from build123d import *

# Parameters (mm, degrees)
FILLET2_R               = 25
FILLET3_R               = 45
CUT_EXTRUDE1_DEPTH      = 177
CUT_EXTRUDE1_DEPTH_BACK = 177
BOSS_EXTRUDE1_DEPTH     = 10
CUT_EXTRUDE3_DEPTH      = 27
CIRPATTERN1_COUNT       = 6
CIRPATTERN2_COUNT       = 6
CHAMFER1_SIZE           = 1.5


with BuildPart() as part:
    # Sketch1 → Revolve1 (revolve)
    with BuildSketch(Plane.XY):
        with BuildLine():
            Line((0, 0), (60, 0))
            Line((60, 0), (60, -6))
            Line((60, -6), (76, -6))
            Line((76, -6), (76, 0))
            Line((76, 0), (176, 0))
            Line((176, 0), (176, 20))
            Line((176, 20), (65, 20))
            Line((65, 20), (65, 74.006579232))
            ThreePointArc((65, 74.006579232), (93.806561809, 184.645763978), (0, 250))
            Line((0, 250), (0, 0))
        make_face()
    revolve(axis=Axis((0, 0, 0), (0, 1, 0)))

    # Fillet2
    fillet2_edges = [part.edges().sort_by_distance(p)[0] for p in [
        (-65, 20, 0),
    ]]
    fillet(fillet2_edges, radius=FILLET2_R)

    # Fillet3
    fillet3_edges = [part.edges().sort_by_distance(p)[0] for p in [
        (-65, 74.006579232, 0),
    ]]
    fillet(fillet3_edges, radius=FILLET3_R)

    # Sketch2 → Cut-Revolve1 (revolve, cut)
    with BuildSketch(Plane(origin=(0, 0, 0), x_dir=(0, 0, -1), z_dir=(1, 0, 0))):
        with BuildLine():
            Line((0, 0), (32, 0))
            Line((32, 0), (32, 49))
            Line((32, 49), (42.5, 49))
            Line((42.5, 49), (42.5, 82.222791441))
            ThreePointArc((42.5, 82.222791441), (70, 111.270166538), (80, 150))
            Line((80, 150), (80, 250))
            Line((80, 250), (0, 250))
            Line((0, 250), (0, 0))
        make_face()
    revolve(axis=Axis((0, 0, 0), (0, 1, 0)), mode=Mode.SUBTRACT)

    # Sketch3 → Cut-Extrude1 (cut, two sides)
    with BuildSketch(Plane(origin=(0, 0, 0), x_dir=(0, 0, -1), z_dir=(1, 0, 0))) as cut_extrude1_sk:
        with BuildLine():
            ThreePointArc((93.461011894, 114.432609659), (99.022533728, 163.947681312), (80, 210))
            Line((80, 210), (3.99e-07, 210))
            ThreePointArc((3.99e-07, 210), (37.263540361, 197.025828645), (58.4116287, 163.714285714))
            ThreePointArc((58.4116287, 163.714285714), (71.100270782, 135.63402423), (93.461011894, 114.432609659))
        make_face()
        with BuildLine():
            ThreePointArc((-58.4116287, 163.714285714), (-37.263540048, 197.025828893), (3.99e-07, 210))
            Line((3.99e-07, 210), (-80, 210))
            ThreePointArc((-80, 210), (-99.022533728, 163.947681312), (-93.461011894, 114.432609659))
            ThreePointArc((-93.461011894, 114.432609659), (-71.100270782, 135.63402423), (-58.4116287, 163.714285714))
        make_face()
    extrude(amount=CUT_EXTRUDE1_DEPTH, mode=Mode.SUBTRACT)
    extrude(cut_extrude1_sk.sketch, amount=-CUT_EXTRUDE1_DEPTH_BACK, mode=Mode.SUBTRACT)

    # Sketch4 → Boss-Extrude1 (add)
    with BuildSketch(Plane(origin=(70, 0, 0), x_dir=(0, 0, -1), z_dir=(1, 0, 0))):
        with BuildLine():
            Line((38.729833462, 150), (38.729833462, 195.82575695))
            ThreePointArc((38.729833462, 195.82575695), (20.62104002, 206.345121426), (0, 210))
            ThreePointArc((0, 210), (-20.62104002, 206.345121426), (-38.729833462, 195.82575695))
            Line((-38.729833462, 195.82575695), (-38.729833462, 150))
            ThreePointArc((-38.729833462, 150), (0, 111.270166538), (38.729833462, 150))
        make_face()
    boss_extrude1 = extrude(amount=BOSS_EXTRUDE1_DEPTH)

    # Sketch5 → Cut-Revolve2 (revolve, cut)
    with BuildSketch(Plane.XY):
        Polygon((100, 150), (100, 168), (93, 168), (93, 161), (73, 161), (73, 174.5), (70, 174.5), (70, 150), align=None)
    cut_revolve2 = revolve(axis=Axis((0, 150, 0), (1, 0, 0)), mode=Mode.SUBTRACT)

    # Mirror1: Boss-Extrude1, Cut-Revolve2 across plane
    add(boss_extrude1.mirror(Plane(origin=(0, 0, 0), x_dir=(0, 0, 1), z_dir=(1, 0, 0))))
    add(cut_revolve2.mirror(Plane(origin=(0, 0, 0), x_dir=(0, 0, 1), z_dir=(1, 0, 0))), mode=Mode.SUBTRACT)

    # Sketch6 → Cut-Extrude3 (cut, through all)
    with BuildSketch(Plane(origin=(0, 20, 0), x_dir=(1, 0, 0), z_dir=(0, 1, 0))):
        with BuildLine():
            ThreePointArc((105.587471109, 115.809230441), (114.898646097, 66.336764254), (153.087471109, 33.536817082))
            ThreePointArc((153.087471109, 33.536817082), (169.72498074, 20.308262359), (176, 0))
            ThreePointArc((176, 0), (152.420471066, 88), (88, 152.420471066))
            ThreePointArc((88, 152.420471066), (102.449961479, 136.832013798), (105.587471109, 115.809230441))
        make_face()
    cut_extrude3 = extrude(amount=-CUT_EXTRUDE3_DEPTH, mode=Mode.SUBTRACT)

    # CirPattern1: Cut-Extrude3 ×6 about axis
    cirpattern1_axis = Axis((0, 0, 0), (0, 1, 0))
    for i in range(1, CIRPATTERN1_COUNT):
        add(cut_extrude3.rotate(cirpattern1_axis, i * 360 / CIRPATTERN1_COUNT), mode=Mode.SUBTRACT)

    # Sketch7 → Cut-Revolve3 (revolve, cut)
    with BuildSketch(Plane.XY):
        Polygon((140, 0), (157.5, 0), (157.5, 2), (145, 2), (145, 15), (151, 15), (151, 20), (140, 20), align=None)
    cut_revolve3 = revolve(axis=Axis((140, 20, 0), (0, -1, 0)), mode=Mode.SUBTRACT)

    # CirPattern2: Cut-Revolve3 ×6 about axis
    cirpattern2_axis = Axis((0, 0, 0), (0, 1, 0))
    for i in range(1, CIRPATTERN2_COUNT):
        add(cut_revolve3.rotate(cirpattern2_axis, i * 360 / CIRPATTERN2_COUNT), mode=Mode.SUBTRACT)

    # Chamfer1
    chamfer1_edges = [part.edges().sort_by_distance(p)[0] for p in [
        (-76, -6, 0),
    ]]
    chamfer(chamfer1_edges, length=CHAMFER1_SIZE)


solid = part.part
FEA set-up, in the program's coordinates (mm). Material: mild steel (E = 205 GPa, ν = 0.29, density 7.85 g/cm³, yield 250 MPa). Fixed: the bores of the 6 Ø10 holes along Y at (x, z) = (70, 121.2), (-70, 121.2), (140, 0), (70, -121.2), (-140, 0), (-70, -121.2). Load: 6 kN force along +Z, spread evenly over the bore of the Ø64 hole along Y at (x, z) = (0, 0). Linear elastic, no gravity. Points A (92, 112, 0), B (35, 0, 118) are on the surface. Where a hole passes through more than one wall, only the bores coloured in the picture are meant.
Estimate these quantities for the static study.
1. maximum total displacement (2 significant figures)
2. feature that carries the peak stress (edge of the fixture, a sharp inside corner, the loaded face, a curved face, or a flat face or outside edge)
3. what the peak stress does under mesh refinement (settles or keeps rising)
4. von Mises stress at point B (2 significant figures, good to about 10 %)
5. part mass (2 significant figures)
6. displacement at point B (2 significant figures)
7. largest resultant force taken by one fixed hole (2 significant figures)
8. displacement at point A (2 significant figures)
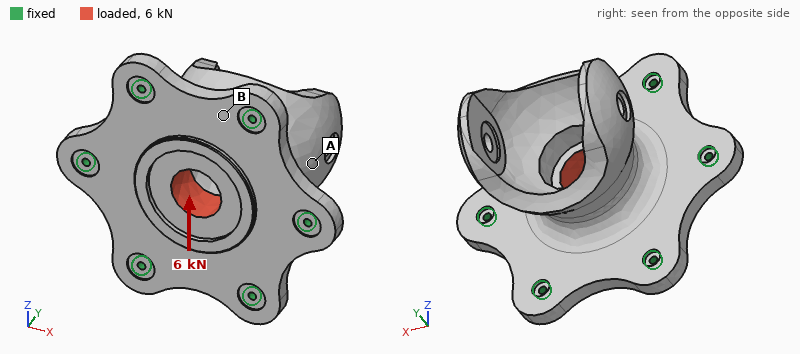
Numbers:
2.0 µm
edge of the fixture
keeps rising
0.69 MPa
23 kg
0.52 µm
1.4 kN
1.3 µm
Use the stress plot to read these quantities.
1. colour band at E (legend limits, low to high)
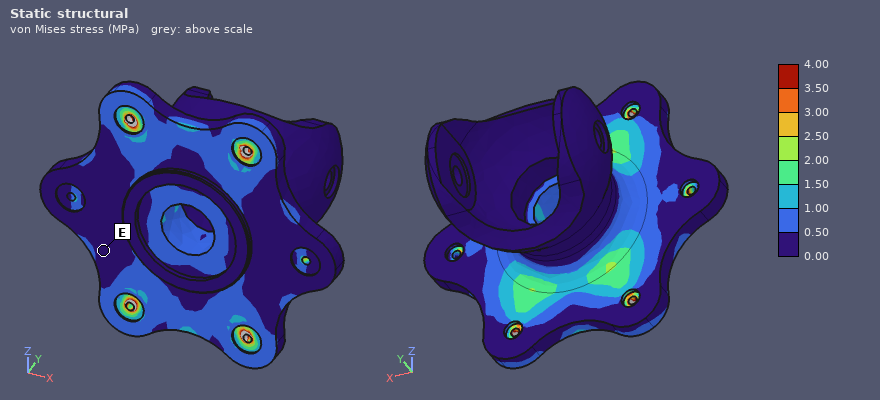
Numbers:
0.00 to 0.50 MPa
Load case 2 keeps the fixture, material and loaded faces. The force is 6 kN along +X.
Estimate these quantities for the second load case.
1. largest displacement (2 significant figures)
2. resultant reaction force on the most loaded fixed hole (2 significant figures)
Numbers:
2.0 µm
1.6 kN
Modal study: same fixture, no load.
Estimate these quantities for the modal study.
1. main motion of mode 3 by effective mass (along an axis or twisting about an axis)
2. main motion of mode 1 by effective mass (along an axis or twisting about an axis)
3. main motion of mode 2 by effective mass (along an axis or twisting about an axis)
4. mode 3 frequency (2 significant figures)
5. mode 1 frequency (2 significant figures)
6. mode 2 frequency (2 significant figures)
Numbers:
along Y
along X
along Z
1200 Hz
990 Hz
1100 Hz
